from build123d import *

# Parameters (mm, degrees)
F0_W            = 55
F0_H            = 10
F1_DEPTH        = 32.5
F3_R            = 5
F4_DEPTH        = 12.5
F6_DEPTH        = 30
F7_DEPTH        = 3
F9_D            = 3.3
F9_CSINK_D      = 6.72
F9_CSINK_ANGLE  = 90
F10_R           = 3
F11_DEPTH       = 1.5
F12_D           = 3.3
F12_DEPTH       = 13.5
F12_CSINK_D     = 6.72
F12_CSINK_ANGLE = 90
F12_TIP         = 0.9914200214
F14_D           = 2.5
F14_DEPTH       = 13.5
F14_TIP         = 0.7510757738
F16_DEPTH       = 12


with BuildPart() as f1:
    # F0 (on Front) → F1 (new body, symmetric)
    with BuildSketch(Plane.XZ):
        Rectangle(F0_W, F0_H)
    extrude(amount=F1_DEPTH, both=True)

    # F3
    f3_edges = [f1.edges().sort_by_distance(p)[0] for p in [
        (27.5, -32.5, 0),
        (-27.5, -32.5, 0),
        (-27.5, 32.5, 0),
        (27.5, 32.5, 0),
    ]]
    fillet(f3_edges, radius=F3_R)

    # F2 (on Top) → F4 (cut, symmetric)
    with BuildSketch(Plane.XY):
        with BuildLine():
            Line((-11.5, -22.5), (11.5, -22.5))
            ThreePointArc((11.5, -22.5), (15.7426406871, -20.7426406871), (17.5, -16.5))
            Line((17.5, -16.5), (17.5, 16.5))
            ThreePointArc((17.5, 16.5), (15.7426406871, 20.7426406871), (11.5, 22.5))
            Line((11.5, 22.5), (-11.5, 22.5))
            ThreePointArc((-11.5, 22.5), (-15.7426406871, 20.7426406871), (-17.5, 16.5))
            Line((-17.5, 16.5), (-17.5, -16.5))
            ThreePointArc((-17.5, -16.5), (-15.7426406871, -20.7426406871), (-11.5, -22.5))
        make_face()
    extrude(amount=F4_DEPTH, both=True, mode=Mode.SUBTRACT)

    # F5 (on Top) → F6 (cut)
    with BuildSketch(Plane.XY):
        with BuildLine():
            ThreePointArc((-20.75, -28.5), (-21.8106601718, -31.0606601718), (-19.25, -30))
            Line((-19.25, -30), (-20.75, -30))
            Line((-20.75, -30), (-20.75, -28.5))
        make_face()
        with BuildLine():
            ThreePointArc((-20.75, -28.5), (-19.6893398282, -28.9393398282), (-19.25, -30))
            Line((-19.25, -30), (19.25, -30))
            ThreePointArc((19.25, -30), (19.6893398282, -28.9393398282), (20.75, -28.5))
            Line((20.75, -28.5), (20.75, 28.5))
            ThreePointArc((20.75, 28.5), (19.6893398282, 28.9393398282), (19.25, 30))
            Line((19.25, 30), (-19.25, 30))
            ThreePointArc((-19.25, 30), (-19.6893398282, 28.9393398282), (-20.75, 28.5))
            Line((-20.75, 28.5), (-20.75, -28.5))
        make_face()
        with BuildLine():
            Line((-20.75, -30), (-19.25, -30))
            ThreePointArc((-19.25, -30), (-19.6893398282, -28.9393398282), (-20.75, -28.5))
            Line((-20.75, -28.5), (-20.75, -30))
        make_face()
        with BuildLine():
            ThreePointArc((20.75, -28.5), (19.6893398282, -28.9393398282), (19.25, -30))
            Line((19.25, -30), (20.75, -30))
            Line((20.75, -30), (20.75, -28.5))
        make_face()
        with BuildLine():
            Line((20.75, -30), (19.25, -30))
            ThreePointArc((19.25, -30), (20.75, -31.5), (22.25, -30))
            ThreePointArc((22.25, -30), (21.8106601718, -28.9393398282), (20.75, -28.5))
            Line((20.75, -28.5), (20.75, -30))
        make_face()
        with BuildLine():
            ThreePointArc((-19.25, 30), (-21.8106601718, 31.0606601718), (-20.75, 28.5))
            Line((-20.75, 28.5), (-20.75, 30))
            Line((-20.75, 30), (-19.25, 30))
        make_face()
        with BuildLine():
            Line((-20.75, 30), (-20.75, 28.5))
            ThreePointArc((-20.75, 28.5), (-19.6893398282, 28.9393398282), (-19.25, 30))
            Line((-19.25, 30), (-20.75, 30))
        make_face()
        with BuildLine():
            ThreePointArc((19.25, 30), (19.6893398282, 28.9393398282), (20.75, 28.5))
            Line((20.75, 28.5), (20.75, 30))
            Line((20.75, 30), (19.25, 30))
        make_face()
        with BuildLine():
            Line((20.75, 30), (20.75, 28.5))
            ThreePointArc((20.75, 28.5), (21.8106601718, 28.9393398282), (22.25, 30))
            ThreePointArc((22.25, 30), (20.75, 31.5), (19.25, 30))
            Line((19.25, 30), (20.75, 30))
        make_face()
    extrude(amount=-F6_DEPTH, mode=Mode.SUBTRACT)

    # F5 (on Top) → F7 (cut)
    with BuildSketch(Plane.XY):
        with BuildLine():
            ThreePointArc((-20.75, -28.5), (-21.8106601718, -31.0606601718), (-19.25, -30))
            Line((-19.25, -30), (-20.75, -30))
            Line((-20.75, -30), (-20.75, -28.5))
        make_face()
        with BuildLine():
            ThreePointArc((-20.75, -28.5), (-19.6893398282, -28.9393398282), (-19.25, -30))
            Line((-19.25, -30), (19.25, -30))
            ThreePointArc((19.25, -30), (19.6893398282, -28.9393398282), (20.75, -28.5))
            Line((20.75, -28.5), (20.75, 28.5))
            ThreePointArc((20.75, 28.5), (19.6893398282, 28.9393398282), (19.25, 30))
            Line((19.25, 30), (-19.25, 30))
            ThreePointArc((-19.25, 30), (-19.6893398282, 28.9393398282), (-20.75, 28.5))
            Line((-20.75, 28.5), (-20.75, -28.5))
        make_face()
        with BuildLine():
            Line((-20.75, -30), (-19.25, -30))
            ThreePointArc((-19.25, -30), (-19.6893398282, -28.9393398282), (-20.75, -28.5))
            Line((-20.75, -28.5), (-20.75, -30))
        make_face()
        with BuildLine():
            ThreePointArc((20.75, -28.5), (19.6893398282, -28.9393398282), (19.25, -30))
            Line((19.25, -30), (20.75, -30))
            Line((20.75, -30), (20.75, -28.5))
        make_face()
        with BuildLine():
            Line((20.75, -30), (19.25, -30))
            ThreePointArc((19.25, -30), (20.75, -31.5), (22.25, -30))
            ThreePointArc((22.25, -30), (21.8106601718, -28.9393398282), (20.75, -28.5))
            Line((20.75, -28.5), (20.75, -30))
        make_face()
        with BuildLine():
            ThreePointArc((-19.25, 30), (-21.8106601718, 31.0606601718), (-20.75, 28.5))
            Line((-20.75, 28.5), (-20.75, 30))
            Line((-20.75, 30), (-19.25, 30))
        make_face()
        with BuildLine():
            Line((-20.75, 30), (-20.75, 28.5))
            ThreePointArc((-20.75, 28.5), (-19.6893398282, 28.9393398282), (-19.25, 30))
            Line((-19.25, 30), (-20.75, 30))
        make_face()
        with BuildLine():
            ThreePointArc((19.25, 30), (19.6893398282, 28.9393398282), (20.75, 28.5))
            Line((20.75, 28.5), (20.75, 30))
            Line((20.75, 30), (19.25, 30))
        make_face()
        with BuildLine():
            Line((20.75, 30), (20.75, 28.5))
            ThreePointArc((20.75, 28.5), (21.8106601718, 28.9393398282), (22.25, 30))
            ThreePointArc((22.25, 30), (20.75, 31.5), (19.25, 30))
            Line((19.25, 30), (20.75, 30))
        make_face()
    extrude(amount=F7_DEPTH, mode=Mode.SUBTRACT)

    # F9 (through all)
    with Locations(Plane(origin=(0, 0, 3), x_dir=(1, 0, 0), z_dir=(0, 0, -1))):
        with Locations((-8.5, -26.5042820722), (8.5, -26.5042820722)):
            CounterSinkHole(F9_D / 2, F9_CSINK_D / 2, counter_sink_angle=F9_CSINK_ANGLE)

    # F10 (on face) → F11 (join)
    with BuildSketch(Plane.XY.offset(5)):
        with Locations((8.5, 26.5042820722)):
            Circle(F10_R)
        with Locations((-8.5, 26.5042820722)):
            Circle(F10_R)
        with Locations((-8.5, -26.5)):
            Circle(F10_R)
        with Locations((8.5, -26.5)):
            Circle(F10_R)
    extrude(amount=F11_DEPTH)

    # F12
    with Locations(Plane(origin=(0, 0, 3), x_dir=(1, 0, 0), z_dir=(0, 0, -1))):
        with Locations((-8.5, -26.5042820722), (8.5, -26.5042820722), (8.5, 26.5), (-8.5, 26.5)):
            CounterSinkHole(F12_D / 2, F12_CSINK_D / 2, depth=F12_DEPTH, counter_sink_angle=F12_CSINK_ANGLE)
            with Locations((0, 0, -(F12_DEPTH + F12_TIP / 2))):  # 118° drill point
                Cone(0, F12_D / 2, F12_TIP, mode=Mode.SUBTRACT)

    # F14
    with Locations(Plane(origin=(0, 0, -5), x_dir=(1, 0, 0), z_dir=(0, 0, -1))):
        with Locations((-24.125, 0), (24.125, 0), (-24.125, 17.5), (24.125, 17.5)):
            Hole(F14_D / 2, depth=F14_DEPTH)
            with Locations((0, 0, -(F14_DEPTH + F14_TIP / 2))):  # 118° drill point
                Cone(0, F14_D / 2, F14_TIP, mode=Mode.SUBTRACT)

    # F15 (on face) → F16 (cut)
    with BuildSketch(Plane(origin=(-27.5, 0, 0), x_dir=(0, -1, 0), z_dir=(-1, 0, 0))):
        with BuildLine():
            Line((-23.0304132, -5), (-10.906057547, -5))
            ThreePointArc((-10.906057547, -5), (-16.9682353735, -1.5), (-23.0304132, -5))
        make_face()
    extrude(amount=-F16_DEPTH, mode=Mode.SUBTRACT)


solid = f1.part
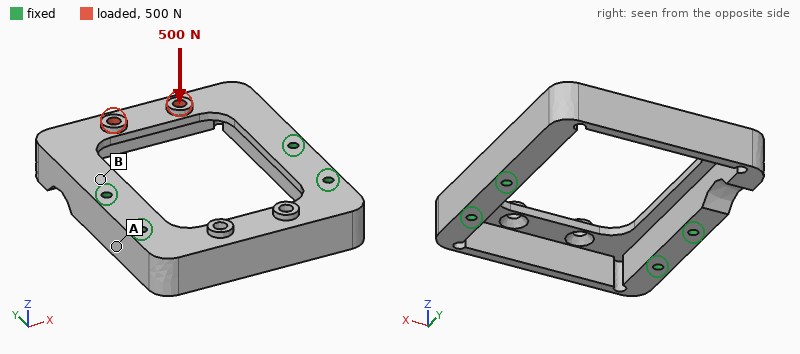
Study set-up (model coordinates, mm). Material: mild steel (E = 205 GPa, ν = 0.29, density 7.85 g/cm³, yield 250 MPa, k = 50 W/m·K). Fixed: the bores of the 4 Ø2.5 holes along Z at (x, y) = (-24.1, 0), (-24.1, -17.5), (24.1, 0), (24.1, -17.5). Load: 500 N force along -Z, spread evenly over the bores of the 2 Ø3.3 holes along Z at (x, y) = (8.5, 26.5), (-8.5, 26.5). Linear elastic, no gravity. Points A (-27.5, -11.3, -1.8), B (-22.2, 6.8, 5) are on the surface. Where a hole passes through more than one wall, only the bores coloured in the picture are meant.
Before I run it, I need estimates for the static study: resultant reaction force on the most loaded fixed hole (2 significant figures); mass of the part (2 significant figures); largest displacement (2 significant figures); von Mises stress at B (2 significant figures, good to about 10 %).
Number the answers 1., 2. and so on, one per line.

1. 330 N
2. 94 g
3. 45 µm
4. 38 MPa
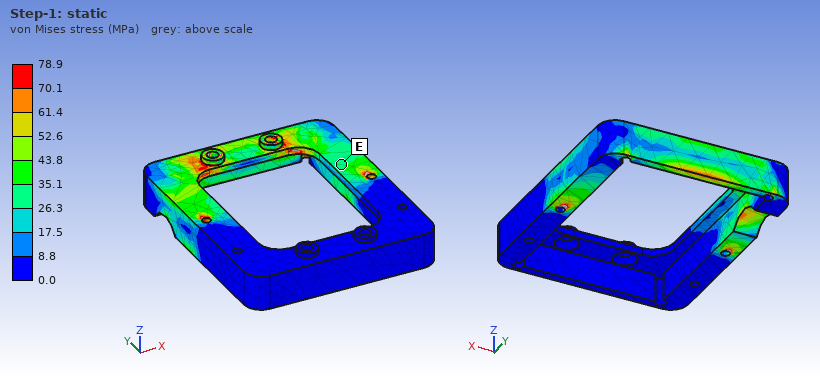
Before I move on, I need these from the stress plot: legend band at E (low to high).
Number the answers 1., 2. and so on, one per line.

1. 26.3 to 35.1 MPa
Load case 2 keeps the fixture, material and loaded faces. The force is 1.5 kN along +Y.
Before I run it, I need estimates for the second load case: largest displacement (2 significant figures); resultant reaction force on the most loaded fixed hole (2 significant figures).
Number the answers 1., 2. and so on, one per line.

1. 30 µm
2. 820 N
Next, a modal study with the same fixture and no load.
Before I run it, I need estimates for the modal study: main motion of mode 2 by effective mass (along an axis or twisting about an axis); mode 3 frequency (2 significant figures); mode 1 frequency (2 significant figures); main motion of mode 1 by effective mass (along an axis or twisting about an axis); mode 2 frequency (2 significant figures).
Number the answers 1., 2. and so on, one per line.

1. along X
2. 7900 Hz
3. 4700 Hz
4. along Z
5. 5700 Hz
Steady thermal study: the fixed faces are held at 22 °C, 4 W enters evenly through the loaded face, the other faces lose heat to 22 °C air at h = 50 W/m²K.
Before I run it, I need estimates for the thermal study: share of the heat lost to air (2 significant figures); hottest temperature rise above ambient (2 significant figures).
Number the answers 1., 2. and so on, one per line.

1. 48 %
2. 25 K
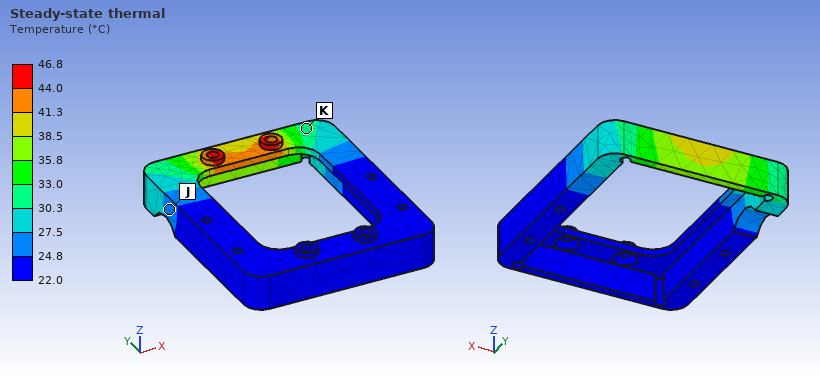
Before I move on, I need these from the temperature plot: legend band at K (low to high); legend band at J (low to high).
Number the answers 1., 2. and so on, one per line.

1. 30.3 to 33.0 °C
2. 24.8 to 27.5 °C
